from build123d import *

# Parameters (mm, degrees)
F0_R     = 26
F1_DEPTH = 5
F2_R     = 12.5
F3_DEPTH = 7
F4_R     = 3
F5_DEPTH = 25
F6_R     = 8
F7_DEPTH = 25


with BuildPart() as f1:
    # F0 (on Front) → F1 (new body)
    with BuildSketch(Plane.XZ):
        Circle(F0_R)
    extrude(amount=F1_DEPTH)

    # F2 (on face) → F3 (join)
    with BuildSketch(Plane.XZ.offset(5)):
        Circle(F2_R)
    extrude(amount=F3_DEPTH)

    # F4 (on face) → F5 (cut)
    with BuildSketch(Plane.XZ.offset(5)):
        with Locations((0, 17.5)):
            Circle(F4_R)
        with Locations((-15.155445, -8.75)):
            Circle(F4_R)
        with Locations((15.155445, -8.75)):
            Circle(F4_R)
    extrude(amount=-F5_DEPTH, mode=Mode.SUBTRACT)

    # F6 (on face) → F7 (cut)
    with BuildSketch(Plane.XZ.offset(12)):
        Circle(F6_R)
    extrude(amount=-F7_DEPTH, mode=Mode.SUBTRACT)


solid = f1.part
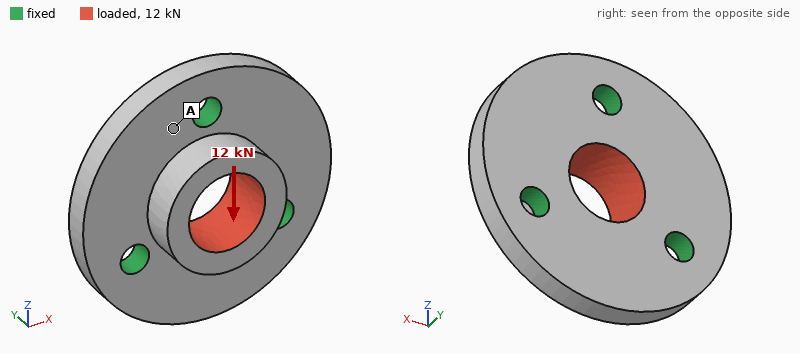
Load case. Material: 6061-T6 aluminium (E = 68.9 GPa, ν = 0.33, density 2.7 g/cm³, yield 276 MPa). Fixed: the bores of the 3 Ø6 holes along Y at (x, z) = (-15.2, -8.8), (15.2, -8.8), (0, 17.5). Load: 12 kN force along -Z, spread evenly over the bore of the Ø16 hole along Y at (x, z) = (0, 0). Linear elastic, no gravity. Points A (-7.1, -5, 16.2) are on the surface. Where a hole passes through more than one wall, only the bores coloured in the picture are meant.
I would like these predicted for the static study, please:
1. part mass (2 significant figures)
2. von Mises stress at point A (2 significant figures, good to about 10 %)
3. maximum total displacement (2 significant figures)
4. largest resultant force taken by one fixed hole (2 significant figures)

30 g
25 MPa
31 µm
4.2 kN
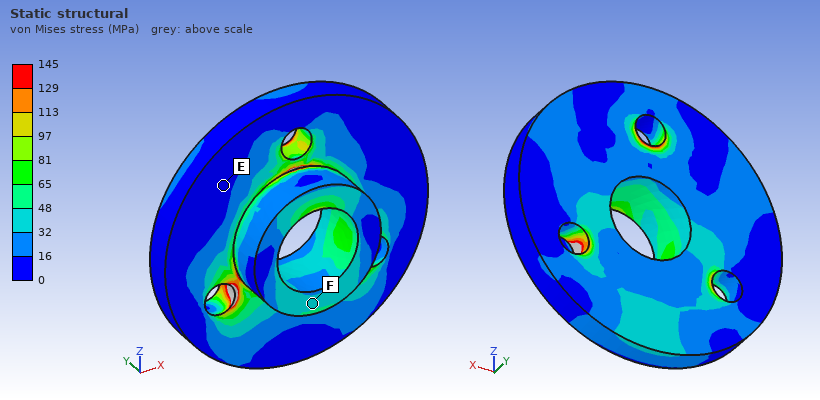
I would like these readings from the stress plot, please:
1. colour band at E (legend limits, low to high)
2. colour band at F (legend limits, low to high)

0 to 16 MPa
32 to 48 MPa
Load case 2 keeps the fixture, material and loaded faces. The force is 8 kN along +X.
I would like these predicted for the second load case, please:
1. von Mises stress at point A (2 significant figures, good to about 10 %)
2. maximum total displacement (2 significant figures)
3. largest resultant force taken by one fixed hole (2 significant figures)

30 MPa
19 µm
2.8 kN
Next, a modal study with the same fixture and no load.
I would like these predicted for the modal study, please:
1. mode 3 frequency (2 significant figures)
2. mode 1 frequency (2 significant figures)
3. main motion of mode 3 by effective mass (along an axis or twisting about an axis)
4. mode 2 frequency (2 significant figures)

17 kHz
16 kHz
along Y
16 kHz
